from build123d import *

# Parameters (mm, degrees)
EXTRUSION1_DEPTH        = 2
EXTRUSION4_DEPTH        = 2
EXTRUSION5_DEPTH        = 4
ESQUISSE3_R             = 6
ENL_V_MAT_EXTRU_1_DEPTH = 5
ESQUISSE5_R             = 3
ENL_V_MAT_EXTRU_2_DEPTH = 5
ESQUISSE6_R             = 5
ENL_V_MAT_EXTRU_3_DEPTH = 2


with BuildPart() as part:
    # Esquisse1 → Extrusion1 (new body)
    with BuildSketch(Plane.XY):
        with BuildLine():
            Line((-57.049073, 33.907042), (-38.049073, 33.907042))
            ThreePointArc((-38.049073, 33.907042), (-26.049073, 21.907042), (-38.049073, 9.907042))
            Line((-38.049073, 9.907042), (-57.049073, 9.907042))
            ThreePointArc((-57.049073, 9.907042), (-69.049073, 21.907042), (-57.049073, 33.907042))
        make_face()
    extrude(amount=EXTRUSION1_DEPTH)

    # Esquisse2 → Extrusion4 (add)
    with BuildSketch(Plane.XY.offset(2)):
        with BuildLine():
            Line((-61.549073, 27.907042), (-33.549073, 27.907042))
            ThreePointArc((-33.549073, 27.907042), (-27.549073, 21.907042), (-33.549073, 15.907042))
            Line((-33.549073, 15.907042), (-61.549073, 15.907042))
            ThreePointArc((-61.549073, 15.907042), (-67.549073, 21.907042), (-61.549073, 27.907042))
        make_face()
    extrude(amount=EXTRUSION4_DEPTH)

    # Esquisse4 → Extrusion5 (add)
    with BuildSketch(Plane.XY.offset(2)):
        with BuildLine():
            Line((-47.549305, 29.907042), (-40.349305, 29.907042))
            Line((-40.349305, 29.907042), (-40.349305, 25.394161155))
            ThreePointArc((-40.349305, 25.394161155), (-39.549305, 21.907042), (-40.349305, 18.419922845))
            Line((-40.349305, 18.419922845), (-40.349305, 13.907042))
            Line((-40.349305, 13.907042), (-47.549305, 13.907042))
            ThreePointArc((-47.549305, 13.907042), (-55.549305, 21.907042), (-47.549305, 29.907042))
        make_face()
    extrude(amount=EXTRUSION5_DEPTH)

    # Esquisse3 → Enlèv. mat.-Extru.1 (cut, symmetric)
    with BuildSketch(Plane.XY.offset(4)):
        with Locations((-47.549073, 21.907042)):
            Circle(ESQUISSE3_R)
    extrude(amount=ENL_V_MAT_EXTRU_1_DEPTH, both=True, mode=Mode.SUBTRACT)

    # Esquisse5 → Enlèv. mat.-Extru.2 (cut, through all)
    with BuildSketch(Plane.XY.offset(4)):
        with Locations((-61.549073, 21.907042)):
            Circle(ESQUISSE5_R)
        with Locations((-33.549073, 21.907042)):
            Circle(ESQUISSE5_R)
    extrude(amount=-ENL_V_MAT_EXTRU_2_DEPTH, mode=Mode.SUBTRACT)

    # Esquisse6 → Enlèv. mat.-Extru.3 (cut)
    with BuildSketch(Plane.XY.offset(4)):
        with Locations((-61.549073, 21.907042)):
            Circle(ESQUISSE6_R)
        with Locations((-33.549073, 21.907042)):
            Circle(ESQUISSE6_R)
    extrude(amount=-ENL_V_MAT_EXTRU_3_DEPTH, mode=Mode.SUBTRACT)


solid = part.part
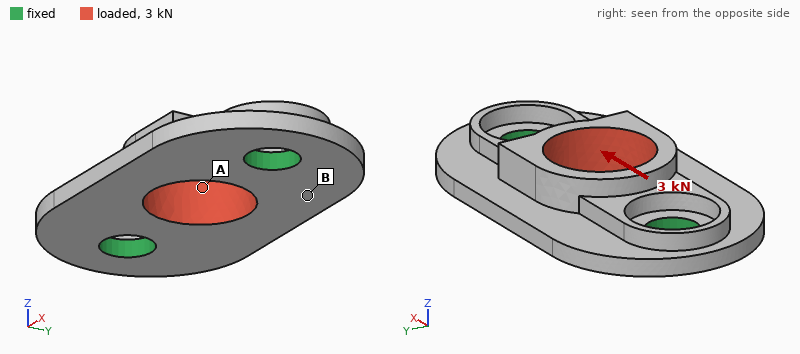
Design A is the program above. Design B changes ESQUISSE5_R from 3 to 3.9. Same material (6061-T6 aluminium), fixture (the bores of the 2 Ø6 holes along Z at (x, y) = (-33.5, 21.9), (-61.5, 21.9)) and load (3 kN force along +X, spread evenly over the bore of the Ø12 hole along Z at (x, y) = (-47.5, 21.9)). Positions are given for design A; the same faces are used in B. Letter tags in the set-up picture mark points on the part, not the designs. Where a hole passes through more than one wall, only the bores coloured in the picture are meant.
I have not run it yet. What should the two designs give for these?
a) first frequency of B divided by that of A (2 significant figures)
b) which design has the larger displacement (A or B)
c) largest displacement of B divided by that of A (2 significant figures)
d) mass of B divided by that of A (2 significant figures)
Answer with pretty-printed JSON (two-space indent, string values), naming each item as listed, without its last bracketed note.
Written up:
{
  "first frequency of B divided by that of A": "1.2",
  "which design has the larger displacement": "A",
  "largest displacement of B divided by that of A": "0.88",
  "mass of B divided by that of A": "0.96"
}
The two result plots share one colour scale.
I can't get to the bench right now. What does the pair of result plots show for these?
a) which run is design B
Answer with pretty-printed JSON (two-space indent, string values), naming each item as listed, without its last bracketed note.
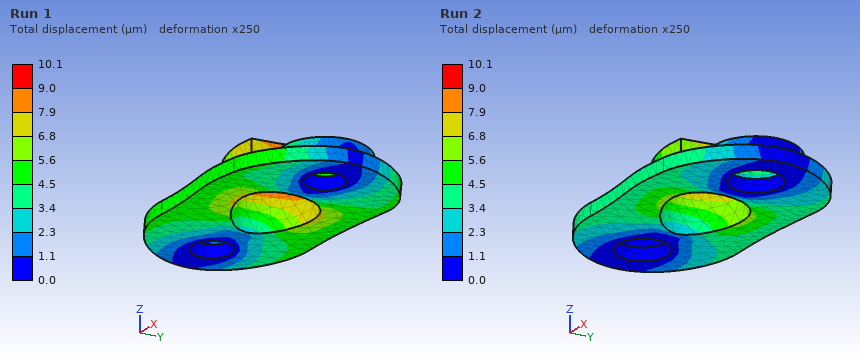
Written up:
{
  "which run is design B": "Run 2"
}
